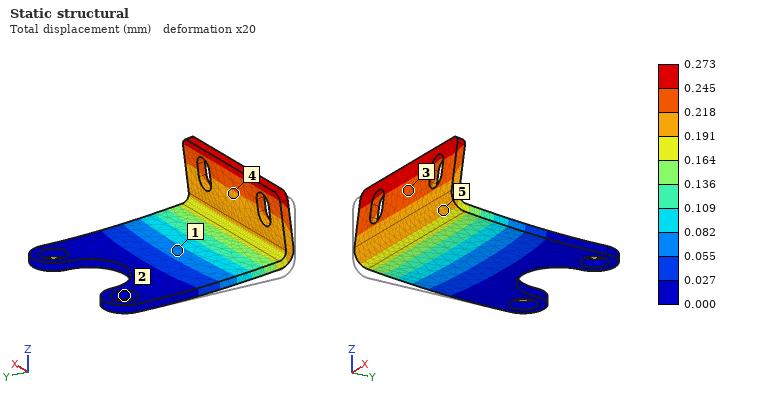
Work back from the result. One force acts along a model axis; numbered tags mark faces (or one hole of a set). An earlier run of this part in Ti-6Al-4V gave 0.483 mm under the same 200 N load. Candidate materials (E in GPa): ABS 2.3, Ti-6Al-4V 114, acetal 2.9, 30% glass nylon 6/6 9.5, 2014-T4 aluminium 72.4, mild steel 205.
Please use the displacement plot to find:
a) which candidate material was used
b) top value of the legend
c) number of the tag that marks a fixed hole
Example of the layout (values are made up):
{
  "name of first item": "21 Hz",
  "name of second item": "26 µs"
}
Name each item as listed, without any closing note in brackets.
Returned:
{
  "which candidate material was used": "mild steel",
  "top value of the legend": "0.273 mm",
  "number of the tag that marks a fixed hole": "2"
}
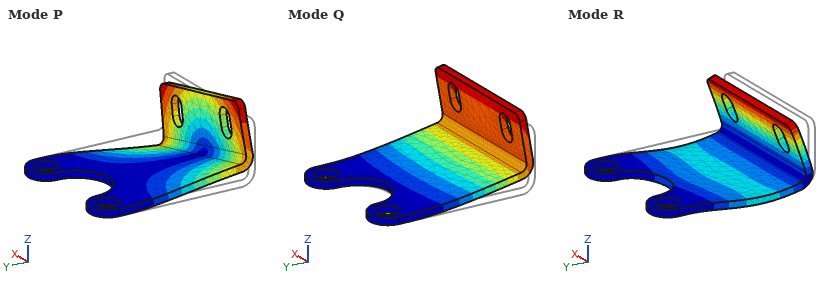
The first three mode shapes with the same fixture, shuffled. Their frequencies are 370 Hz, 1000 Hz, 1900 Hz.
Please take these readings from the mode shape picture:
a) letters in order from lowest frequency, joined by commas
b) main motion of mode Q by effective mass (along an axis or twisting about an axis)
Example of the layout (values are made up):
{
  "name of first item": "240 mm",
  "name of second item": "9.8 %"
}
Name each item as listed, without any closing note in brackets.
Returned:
{
  "letters in order from lowest frequency, joined by commas": "Q, P, R",
  "main motion of mode Q by effective mass": "along Z"
}
